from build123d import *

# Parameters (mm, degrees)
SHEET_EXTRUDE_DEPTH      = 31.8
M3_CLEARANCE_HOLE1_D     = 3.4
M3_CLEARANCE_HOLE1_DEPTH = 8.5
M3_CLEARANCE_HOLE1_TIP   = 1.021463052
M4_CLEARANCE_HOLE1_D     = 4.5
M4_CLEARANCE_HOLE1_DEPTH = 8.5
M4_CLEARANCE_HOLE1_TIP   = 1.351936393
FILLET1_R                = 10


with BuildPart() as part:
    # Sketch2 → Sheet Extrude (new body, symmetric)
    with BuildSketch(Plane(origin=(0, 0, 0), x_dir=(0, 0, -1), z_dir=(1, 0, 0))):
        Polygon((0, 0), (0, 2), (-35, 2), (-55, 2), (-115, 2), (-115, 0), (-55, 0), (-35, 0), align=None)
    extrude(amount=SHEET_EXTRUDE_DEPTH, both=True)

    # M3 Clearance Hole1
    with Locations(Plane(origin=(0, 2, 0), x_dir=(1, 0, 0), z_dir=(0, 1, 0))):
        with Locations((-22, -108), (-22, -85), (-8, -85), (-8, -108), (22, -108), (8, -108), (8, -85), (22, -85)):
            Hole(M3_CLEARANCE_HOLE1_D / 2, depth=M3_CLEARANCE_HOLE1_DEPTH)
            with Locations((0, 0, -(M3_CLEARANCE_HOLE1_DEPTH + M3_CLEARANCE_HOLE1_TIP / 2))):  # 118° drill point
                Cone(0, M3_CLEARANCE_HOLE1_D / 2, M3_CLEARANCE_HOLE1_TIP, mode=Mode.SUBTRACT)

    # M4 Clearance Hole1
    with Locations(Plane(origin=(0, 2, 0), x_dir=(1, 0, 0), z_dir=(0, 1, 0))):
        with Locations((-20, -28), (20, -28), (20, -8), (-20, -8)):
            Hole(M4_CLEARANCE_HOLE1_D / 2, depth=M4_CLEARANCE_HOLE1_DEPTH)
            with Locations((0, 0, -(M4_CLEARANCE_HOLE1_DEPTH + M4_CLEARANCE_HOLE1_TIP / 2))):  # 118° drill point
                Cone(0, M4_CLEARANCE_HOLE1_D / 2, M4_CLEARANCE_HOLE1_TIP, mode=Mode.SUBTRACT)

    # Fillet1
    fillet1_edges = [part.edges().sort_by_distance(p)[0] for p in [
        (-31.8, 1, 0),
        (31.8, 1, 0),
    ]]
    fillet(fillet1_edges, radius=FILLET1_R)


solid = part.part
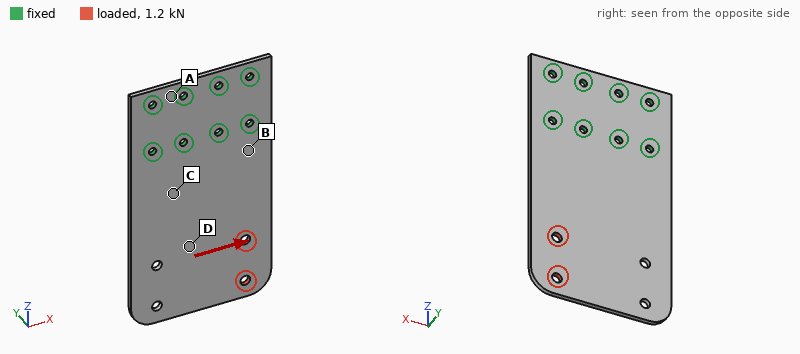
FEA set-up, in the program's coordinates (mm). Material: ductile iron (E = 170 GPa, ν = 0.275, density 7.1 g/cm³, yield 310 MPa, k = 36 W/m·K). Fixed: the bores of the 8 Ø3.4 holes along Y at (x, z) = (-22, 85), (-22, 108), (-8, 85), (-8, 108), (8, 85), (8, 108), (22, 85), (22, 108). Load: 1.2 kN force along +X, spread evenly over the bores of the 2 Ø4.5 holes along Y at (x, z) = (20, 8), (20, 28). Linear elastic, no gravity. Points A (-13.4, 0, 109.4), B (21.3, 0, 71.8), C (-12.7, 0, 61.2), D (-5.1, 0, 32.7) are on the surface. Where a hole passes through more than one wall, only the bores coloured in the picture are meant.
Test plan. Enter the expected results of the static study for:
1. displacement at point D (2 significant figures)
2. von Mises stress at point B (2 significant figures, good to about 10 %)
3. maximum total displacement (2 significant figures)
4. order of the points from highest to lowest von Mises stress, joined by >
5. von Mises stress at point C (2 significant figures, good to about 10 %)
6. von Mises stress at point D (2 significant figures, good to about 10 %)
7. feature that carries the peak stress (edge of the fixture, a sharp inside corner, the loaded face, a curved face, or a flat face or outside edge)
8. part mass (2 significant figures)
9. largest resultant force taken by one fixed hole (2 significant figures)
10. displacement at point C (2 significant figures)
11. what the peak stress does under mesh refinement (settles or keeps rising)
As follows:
22 µm
38 MPa
41 µm
B > C > D > A
27 MPa
21 MPa
edge of the fixture
100 g
1.3 kN
8.4 µm
keeps rising
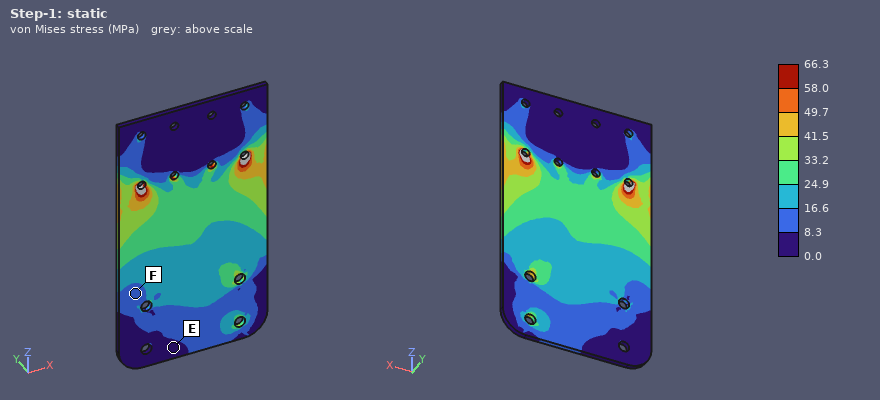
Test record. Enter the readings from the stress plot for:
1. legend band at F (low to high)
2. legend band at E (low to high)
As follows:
8.3 to 16.6 MPa
0.0 to 8.3 MPa
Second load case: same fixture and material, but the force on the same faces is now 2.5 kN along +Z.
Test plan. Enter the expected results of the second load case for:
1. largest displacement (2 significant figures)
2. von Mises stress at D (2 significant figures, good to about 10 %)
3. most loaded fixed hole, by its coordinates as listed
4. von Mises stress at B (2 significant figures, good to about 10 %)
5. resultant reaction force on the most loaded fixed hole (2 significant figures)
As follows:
33 µm
8.7 MPa
(22, 85)
48 MPa
1.4 kN
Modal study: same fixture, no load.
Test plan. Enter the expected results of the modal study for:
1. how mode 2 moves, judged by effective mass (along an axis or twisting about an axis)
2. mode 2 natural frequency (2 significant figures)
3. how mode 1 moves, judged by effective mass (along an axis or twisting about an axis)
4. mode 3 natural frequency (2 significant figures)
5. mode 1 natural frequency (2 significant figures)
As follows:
twisting about Z
710 Hz
along Y
1400 Hz
230 Hz
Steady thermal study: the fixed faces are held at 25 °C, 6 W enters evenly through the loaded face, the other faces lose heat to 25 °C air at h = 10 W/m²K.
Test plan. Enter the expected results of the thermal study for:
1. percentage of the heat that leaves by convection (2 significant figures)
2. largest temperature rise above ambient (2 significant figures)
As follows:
53 %
76 K
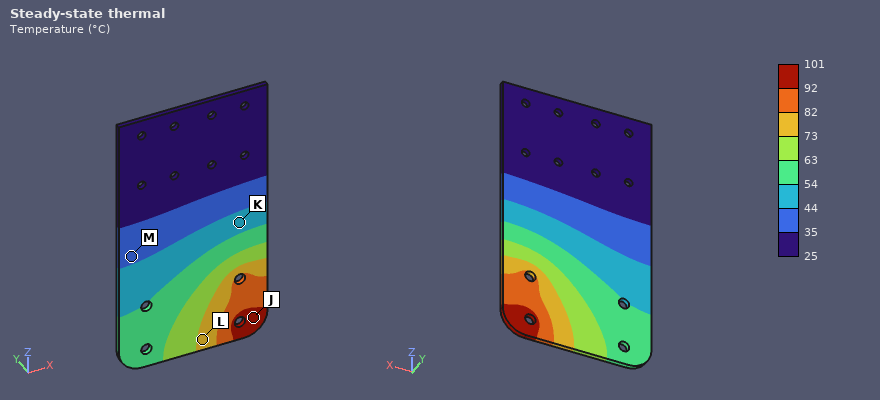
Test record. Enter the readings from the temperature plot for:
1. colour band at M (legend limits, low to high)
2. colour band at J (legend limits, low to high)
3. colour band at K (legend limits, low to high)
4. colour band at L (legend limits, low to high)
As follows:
35 to 44 °C
92 to 101 °C
44 to 54 °C
73 to 82 °C
